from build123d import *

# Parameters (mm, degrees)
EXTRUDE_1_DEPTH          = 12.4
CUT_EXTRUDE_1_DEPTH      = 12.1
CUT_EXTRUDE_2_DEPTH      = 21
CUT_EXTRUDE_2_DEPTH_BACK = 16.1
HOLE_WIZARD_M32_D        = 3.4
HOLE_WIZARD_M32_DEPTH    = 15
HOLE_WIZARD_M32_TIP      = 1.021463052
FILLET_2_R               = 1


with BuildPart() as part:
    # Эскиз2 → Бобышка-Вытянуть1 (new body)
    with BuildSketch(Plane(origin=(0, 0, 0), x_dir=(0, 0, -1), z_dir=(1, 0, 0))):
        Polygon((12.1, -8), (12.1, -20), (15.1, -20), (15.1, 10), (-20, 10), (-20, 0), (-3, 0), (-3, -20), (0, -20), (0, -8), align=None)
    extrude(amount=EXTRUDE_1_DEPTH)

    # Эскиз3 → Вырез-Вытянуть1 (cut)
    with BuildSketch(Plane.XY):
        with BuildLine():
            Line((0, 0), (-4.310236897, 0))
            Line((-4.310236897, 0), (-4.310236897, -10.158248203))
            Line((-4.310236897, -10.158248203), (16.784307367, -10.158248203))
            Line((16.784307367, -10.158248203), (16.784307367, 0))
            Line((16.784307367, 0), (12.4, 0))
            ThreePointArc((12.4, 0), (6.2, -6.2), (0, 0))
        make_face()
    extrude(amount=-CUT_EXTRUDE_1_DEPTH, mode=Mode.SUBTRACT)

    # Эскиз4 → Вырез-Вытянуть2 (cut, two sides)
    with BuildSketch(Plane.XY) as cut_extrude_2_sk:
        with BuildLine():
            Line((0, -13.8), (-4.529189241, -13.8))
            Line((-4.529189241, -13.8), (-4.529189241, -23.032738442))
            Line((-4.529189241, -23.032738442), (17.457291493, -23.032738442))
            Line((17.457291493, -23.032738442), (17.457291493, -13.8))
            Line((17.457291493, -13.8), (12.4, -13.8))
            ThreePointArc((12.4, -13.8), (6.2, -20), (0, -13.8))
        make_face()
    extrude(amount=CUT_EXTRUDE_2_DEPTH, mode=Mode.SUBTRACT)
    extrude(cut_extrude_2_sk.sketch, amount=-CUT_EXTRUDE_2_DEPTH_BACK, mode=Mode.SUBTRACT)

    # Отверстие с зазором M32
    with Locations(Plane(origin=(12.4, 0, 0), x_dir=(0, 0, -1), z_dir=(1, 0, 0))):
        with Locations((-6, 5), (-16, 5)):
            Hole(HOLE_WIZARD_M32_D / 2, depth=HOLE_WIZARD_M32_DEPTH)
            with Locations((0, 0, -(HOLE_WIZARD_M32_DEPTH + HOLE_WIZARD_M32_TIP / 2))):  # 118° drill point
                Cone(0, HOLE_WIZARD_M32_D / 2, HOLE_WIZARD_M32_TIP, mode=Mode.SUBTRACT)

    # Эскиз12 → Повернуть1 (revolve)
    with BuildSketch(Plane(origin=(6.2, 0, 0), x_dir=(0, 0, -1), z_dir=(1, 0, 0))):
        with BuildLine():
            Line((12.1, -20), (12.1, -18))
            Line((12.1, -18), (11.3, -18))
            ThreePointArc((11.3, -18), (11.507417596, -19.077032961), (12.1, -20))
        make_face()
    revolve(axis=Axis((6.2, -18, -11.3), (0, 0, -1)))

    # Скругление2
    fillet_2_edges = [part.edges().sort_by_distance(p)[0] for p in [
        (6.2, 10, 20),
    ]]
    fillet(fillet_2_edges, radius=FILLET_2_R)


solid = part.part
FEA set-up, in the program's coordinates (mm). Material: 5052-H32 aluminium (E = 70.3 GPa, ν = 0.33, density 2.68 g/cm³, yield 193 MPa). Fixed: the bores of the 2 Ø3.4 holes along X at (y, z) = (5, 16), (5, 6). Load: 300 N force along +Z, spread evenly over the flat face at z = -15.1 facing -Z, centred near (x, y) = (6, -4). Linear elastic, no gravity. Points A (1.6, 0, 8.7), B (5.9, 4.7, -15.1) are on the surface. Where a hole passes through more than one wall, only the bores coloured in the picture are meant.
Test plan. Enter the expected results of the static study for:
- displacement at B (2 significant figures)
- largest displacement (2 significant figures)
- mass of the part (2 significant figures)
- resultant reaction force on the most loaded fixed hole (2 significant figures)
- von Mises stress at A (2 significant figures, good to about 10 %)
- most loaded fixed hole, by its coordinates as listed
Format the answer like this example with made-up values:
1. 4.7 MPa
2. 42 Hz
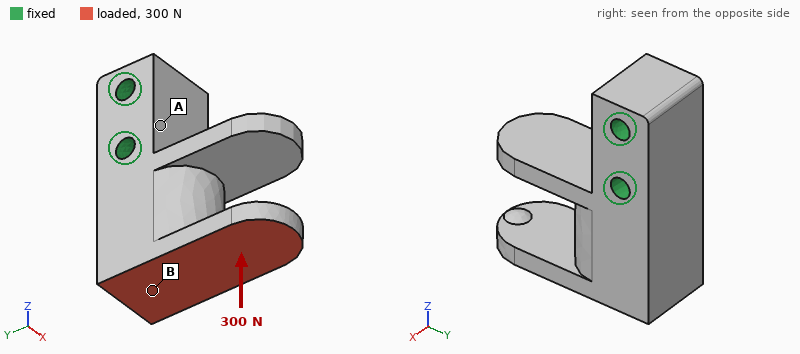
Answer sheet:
1. 7.4 µm
2. 48 µm
3. 17 g
4. 290 N
5. 6.5 MPa
6. (5, 6)
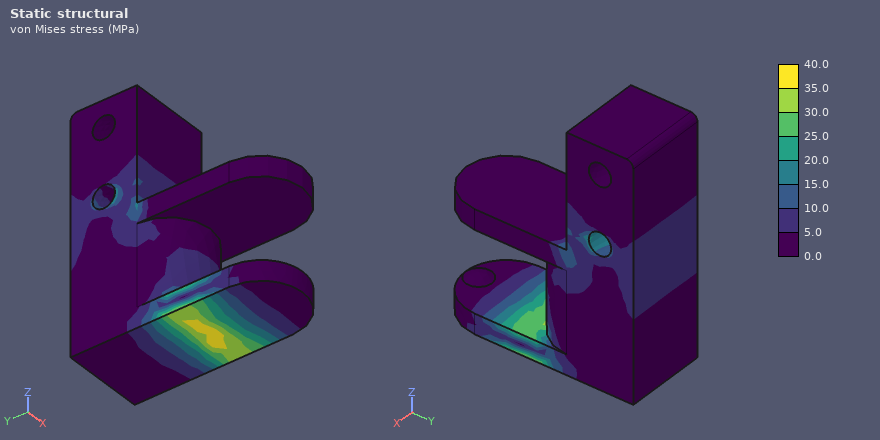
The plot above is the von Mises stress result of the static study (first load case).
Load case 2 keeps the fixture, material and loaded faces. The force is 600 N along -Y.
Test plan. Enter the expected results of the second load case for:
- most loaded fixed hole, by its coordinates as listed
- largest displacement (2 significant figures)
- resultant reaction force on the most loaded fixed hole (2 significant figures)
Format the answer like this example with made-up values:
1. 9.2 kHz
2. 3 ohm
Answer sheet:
1. (5, 6)
2. 72 µm
3. 1.1 kN
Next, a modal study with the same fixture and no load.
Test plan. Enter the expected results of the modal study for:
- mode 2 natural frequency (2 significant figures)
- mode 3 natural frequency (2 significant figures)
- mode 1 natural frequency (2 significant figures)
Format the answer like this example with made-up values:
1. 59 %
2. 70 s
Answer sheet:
1. 11 kHz
2. 11 kHz
3. 7400 Hz
